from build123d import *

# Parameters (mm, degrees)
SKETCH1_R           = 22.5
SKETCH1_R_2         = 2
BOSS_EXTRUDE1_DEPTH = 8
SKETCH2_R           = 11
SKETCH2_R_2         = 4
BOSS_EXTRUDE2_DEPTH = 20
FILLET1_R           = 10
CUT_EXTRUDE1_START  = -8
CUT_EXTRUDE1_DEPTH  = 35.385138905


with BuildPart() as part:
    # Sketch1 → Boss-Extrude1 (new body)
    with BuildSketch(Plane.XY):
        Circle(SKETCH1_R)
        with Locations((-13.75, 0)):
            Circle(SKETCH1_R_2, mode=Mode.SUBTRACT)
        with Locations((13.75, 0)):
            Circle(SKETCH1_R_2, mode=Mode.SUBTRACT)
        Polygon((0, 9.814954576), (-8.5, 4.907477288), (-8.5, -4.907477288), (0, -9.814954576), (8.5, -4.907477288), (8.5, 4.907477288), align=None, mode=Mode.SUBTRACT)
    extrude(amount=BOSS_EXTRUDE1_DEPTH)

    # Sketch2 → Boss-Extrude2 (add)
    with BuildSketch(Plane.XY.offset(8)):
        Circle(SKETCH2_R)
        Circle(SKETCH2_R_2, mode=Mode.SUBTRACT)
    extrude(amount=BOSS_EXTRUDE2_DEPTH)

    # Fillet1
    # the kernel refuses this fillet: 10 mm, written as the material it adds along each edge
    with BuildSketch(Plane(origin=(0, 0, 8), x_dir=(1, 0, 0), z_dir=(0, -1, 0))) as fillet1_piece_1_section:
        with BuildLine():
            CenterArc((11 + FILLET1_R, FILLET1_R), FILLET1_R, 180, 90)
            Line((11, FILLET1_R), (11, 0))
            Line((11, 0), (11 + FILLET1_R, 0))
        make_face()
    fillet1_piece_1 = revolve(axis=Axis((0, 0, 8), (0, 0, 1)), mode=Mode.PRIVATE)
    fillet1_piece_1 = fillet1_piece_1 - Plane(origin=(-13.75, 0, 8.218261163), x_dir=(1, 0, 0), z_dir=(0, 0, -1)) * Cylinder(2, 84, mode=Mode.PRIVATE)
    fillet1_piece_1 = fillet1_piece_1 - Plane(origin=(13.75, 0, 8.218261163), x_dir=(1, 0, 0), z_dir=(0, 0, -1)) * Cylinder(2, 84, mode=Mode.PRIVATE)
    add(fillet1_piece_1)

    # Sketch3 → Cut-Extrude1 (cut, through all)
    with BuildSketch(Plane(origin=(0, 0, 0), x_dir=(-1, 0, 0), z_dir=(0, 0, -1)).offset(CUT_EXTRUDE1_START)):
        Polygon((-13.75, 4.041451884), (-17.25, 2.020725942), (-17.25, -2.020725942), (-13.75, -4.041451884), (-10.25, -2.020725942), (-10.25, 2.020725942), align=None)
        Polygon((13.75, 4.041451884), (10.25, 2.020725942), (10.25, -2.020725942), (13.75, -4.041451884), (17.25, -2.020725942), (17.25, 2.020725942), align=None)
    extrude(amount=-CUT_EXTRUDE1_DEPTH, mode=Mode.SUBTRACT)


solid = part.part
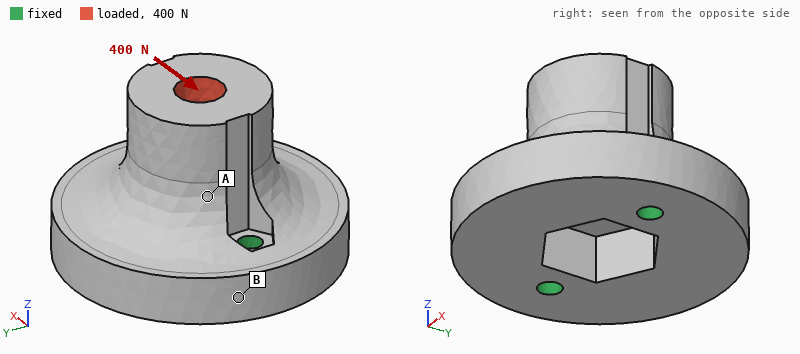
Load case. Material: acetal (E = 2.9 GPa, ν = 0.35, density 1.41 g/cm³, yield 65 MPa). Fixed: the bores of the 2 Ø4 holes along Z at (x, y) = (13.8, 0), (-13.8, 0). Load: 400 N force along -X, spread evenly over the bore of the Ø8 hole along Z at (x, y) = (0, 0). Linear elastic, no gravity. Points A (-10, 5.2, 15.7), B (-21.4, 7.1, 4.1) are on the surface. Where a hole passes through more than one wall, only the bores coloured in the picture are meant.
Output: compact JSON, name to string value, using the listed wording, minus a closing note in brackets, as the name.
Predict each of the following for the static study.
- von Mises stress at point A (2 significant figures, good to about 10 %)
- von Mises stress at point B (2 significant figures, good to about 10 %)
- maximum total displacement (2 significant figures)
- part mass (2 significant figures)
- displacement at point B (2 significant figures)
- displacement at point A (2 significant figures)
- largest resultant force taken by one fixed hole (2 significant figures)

{"von Mises stress at point A": "2.3 MPa", "von Mises stress at point B": "0.78 MPa", "maximum total displacement": "39 µm", "part mass": "26 g", "displacement at point B": "8.4 µm", "displacement at point A": "21 µm", "largest resultant force taken by one fixed hole": "270 N"}
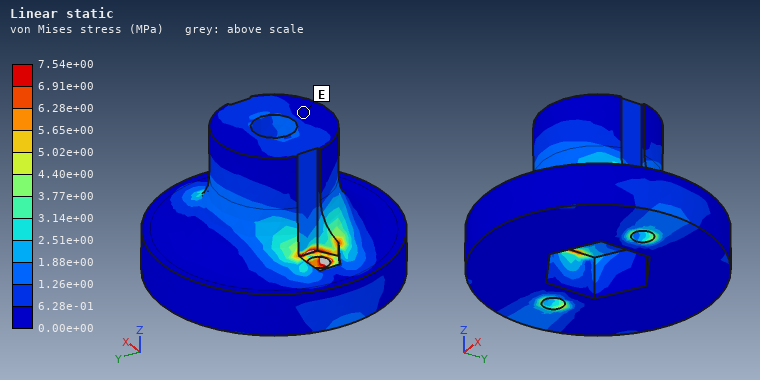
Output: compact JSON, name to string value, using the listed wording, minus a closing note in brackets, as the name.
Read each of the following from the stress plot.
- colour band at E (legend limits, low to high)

{"colour band at E": "0.00e+00 to 6.28e-01 MPa"}
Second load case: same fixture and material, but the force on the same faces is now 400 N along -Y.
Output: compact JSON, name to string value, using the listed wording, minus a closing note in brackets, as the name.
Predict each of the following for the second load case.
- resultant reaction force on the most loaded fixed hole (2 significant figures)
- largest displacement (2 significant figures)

{"resultant reaction force on the most loaded fixed hole": "200 N", "largest displacement": "0.15 mm"}
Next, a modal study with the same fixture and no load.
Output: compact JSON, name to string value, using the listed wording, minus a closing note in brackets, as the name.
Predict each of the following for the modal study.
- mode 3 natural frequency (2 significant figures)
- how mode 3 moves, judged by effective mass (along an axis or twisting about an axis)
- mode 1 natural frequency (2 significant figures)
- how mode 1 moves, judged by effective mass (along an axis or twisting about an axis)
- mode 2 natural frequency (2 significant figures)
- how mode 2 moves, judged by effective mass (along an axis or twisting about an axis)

{"mode 3 natural frequency": "5800 Hz", "how mode 3 moves, judged by effective mass": "along X", "mode 1 natural frequency": "2400 Hz", "how mode 1 moves, judged by effective mass": "along Y", "mode 2 natural frequency": "5200 Hz", "how mode 2 moves, judged by effective mass": "along Z"}
